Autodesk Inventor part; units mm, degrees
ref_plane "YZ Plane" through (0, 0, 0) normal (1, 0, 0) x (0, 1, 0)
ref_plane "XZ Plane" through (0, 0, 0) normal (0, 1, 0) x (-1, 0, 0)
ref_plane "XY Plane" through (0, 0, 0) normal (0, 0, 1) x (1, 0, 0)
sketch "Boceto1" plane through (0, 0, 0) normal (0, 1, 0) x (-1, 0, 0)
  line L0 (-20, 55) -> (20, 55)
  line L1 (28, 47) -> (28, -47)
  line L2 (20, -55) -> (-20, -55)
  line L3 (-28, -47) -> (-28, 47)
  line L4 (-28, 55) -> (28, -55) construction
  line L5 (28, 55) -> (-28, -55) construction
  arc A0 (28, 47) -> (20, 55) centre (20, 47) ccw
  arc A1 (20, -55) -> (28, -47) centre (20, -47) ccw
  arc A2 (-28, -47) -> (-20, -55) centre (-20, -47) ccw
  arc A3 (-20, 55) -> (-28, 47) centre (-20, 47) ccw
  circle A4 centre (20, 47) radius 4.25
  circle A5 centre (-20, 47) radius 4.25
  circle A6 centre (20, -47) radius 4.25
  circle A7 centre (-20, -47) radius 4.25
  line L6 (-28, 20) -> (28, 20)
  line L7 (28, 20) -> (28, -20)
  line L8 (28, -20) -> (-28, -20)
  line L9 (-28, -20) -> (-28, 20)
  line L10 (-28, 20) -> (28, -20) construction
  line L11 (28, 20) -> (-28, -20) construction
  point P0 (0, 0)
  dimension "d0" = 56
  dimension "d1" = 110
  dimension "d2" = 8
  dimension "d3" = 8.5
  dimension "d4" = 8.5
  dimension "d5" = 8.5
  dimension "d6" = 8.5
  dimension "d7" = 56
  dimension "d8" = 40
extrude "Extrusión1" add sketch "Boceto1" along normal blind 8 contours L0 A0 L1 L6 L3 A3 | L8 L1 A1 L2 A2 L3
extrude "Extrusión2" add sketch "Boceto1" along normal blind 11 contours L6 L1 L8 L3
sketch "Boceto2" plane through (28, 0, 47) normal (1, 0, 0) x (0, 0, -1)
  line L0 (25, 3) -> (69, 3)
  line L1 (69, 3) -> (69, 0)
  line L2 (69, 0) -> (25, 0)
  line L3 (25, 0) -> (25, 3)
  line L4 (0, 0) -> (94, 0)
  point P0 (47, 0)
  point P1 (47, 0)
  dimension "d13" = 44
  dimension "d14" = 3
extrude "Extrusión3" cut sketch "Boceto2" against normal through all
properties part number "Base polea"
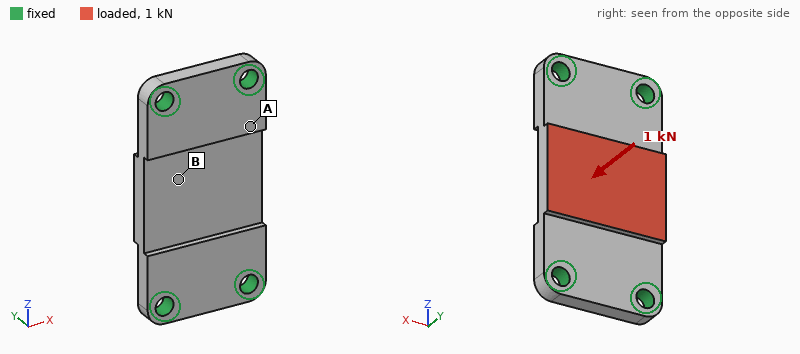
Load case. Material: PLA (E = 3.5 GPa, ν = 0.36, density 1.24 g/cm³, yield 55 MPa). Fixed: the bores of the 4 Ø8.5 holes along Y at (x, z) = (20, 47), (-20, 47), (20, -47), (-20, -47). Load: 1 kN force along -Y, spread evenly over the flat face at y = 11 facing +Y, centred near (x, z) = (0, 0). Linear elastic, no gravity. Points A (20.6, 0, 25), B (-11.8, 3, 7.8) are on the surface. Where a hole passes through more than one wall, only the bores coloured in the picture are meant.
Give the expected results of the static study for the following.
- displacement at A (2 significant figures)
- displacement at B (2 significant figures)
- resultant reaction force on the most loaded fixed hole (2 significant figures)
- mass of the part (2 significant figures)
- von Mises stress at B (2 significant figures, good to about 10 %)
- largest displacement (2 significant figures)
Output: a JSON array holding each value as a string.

["0.20 mm", "0.34 mm", "520 N", "57 g", "5.3 MPa", "0.39 mm"]
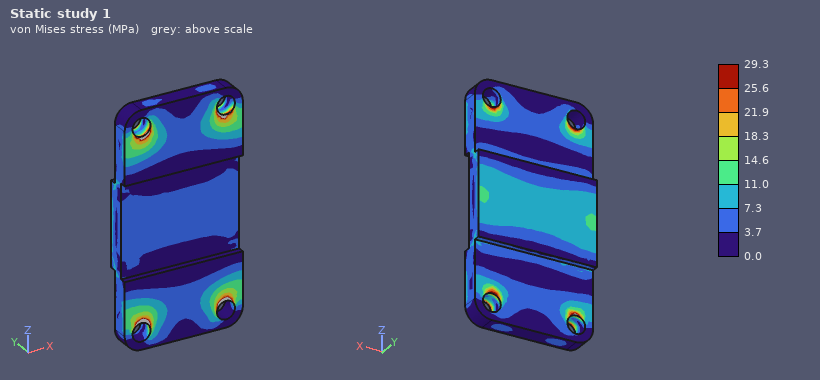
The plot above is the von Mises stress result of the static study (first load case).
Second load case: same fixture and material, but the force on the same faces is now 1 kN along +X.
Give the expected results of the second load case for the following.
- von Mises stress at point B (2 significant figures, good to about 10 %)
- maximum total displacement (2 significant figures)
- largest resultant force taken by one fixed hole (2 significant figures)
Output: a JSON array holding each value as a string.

["1.0 MPa", "0.16 mm", "420 N"]
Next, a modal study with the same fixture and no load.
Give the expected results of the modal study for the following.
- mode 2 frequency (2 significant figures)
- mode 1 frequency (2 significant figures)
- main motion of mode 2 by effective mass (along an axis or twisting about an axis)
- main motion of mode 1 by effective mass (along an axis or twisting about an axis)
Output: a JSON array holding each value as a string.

["2300 Hz", "1700 Hz", "twisting about Z", "along Y"]
